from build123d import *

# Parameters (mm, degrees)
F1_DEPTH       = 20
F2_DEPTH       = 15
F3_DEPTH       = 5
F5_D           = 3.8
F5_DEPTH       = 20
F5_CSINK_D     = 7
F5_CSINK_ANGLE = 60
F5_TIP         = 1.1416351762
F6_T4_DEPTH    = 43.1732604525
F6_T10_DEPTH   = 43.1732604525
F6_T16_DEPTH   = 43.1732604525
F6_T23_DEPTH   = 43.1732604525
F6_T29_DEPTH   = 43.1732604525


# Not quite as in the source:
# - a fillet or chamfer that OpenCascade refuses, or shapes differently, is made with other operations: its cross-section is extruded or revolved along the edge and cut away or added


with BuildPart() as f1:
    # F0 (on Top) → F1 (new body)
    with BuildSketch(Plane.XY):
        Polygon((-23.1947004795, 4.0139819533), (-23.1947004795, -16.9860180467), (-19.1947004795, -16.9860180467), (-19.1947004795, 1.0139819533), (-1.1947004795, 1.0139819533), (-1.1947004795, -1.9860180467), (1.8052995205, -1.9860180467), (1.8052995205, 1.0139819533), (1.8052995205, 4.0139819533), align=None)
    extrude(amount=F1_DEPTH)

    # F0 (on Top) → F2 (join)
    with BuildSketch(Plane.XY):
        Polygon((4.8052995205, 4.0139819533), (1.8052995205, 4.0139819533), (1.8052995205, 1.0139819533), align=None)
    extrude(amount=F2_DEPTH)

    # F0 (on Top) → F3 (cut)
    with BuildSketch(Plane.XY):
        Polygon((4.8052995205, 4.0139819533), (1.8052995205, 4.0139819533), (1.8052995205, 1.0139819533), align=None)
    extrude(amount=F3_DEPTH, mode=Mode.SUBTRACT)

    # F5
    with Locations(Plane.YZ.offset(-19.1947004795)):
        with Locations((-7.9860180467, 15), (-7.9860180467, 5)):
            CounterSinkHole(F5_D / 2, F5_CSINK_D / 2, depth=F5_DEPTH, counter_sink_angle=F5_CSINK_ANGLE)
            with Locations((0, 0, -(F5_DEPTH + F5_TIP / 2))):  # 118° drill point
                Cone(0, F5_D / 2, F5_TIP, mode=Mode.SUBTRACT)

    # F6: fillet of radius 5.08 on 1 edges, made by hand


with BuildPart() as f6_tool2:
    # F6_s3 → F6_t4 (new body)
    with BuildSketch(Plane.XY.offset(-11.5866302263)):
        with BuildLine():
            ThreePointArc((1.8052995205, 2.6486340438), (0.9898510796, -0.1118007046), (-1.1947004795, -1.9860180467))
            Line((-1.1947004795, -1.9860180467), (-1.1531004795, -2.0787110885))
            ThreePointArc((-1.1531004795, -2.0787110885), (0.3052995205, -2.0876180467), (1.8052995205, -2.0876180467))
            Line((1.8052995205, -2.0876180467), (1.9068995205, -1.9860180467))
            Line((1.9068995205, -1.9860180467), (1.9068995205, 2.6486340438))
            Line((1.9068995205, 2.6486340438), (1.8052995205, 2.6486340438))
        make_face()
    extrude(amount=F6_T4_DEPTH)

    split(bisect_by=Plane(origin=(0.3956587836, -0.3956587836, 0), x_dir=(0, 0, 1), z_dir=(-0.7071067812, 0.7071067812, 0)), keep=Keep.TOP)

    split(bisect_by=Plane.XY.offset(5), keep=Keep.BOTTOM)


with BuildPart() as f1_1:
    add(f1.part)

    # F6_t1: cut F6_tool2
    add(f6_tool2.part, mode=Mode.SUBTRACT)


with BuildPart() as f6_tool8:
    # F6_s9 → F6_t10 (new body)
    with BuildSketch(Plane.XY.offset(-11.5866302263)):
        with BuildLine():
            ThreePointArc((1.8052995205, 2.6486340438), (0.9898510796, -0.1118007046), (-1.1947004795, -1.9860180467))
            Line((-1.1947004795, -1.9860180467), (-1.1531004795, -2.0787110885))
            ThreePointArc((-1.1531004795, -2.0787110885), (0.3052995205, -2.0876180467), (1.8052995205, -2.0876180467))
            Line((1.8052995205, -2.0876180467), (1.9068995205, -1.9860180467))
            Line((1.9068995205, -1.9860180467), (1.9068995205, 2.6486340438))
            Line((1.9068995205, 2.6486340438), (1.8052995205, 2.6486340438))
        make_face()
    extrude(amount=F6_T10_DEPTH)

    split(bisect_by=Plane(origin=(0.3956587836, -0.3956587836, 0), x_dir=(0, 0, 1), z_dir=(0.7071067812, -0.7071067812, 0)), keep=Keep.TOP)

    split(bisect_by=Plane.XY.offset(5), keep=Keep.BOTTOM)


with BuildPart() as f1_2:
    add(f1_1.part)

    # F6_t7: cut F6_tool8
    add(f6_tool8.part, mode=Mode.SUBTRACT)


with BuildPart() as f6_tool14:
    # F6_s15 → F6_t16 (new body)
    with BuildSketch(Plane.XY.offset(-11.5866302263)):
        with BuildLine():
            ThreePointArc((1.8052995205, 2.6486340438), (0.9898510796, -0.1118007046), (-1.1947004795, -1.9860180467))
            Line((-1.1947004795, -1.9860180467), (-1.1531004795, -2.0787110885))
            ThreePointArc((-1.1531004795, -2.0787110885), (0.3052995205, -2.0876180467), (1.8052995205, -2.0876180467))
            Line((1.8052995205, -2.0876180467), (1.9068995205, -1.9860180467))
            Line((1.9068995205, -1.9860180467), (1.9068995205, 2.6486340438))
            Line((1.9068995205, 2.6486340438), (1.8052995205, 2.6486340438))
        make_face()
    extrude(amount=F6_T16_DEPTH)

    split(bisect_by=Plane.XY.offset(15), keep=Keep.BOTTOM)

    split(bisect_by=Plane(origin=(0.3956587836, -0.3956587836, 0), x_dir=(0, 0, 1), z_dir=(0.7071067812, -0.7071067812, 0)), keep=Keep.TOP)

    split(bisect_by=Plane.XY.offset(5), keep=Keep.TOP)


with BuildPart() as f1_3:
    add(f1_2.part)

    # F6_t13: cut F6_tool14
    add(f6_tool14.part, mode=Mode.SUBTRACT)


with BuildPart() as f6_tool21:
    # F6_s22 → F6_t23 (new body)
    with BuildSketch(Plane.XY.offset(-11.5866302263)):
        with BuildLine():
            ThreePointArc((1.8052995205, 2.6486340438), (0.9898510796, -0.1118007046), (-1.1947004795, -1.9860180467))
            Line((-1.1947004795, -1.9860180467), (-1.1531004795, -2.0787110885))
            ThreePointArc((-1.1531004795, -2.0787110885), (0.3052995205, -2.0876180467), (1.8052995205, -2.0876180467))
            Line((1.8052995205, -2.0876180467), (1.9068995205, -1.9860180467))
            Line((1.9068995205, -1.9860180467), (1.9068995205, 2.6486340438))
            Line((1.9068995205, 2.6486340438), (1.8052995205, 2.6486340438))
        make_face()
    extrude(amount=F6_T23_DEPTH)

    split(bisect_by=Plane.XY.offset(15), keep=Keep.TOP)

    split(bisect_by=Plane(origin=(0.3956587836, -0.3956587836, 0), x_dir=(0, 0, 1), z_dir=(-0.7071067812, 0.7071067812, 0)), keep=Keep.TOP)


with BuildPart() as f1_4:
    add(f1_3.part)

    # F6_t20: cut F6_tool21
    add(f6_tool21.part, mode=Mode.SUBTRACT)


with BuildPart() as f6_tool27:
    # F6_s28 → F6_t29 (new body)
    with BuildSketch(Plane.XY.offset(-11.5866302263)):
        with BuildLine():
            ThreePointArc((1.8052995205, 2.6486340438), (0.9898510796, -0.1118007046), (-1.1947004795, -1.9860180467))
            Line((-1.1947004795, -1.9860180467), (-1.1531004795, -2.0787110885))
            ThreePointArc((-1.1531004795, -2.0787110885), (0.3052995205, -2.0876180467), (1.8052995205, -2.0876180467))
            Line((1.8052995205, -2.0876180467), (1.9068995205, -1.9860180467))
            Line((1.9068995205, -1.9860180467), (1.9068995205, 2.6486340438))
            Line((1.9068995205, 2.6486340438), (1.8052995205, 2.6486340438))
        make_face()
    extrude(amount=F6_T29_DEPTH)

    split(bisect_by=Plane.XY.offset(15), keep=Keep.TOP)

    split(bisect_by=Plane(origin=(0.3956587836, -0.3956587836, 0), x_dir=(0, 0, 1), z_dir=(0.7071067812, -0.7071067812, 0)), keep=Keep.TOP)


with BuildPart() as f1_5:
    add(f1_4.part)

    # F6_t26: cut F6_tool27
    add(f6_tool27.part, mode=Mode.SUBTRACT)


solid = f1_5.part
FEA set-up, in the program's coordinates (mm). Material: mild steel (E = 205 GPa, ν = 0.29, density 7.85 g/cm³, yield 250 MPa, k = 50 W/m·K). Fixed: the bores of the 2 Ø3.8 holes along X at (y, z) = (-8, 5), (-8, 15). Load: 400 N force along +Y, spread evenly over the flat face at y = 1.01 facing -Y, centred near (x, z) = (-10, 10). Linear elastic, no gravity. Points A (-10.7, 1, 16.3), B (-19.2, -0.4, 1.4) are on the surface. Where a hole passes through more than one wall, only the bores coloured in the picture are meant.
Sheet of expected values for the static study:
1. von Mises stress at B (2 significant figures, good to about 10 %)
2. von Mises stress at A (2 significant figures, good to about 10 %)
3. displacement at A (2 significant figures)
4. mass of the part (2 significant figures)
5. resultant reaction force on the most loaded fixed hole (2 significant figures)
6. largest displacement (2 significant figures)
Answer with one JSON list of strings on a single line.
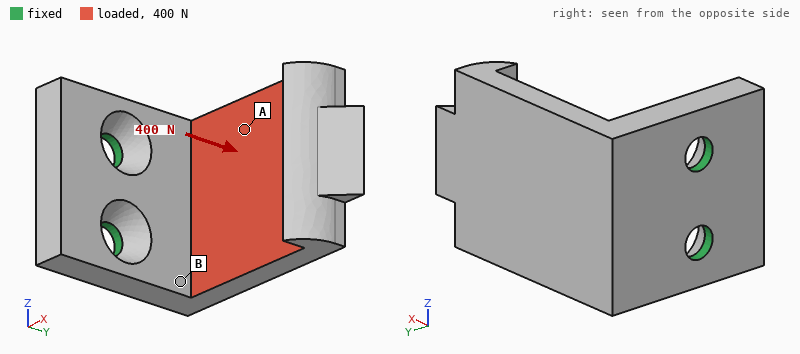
["88 MPa", "34 MPa", "0.053 mm", "23 g", "200 N", "0.15 mm"]
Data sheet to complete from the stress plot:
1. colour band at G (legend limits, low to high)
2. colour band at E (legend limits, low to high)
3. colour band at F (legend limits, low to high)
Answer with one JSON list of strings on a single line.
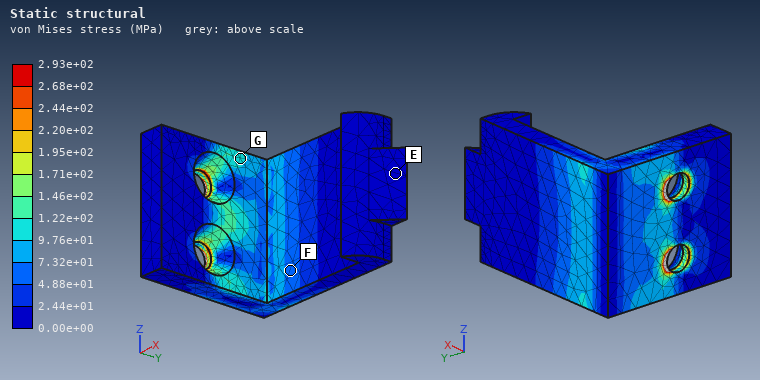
["9.76e+01 to 1.22e+02 MPa", "0.00e+00 to 2.44e+01 MPa", "4.88e+01 to 7.32e+01 MPa"]
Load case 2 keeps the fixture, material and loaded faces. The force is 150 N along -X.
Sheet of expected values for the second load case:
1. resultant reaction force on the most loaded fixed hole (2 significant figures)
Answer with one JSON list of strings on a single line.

["76 N"]
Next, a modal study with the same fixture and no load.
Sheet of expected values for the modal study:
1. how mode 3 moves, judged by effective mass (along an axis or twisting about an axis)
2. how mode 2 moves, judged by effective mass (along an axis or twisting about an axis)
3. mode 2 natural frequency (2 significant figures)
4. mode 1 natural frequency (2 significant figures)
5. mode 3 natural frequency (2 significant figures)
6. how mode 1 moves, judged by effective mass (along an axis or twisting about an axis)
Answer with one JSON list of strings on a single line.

["along X", "along Z", "5600 Hz", "2700 Hz", "8900 Hz", "along Y"]
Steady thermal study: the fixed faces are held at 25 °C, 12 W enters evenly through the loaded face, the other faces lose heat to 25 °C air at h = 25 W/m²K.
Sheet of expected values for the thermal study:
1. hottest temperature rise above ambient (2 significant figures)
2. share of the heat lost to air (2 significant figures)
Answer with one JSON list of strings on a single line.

["65 K", "13 %"]
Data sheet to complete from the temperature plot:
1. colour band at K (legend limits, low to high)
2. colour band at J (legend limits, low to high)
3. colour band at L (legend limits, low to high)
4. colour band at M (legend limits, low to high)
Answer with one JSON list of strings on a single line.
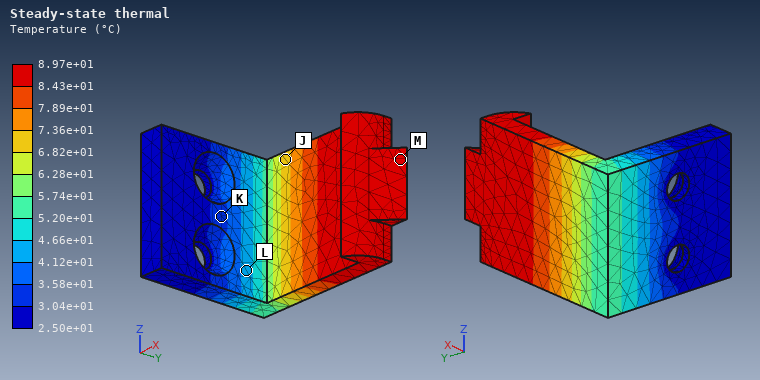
["3.04e+01 to 3.58e+01 °C", "6.82e+01 to 7.36e+01 °C", "4.12e+01 to 4.66e+01 °C", "8.43e+01 to 8.97e+01 °C"]
